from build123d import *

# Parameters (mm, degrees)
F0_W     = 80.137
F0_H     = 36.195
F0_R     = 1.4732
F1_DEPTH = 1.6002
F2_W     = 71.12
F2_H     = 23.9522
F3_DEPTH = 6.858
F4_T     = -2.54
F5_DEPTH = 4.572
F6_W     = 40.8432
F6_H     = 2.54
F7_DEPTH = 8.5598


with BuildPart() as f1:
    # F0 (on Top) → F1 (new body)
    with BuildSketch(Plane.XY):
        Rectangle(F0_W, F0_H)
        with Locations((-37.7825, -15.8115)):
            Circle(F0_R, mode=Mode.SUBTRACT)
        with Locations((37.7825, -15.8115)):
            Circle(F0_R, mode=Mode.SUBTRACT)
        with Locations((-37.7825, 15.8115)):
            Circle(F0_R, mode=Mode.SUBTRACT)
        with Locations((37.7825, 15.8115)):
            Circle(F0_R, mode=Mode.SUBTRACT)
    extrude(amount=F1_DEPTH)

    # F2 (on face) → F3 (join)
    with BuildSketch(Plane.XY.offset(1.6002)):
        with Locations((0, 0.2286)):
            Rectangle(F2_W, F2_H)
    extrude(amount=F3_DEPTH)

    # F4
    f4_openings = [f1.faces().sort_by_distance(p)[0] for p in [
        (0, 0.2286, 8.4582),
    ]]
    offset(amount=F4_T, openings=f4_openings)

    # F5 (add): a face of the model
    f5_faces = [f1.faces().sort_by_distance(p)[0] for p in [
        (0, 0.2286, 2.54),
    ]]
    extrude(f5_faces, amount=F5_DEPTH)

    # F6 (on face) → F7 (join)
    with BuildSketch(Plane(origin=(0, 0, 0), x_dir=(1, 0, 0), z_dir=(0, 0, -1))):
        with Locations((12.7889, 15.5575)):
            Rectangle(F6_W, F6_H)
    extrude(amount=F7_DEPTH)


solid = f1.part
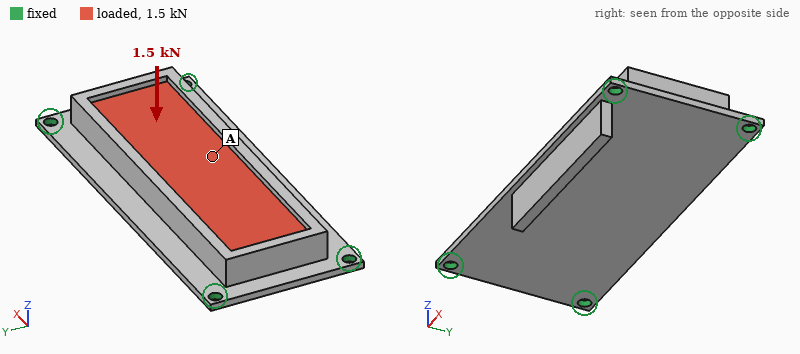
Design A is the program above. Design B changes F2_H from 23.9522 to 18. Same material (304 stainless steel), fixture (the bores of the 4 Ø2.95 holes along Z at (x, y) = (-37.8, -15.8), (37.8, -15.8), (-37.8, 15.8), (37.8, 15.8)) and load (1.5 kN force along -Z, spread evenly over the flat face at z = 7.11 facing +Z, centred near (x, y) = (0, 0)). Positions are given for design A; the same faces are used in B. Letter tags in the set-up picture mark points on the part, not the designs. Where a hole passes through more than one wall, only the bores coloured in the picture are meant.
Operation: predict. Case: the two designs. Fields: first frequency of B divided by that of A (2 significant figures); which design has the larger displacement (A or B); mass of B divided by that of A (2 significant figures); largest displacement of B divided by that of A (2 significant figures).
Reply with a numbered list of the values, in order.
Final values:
1. 0.86
2. B
3. 0.85
4. 1.6
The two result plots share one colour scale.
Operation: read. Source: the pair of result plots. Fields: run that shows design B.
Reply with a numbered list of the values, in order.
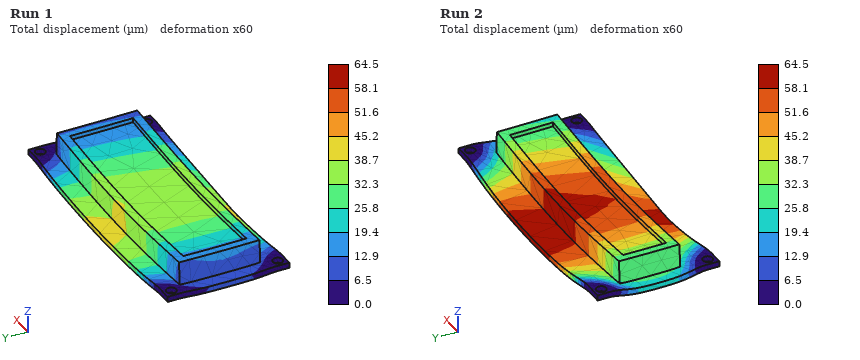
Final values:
1. Run 2
